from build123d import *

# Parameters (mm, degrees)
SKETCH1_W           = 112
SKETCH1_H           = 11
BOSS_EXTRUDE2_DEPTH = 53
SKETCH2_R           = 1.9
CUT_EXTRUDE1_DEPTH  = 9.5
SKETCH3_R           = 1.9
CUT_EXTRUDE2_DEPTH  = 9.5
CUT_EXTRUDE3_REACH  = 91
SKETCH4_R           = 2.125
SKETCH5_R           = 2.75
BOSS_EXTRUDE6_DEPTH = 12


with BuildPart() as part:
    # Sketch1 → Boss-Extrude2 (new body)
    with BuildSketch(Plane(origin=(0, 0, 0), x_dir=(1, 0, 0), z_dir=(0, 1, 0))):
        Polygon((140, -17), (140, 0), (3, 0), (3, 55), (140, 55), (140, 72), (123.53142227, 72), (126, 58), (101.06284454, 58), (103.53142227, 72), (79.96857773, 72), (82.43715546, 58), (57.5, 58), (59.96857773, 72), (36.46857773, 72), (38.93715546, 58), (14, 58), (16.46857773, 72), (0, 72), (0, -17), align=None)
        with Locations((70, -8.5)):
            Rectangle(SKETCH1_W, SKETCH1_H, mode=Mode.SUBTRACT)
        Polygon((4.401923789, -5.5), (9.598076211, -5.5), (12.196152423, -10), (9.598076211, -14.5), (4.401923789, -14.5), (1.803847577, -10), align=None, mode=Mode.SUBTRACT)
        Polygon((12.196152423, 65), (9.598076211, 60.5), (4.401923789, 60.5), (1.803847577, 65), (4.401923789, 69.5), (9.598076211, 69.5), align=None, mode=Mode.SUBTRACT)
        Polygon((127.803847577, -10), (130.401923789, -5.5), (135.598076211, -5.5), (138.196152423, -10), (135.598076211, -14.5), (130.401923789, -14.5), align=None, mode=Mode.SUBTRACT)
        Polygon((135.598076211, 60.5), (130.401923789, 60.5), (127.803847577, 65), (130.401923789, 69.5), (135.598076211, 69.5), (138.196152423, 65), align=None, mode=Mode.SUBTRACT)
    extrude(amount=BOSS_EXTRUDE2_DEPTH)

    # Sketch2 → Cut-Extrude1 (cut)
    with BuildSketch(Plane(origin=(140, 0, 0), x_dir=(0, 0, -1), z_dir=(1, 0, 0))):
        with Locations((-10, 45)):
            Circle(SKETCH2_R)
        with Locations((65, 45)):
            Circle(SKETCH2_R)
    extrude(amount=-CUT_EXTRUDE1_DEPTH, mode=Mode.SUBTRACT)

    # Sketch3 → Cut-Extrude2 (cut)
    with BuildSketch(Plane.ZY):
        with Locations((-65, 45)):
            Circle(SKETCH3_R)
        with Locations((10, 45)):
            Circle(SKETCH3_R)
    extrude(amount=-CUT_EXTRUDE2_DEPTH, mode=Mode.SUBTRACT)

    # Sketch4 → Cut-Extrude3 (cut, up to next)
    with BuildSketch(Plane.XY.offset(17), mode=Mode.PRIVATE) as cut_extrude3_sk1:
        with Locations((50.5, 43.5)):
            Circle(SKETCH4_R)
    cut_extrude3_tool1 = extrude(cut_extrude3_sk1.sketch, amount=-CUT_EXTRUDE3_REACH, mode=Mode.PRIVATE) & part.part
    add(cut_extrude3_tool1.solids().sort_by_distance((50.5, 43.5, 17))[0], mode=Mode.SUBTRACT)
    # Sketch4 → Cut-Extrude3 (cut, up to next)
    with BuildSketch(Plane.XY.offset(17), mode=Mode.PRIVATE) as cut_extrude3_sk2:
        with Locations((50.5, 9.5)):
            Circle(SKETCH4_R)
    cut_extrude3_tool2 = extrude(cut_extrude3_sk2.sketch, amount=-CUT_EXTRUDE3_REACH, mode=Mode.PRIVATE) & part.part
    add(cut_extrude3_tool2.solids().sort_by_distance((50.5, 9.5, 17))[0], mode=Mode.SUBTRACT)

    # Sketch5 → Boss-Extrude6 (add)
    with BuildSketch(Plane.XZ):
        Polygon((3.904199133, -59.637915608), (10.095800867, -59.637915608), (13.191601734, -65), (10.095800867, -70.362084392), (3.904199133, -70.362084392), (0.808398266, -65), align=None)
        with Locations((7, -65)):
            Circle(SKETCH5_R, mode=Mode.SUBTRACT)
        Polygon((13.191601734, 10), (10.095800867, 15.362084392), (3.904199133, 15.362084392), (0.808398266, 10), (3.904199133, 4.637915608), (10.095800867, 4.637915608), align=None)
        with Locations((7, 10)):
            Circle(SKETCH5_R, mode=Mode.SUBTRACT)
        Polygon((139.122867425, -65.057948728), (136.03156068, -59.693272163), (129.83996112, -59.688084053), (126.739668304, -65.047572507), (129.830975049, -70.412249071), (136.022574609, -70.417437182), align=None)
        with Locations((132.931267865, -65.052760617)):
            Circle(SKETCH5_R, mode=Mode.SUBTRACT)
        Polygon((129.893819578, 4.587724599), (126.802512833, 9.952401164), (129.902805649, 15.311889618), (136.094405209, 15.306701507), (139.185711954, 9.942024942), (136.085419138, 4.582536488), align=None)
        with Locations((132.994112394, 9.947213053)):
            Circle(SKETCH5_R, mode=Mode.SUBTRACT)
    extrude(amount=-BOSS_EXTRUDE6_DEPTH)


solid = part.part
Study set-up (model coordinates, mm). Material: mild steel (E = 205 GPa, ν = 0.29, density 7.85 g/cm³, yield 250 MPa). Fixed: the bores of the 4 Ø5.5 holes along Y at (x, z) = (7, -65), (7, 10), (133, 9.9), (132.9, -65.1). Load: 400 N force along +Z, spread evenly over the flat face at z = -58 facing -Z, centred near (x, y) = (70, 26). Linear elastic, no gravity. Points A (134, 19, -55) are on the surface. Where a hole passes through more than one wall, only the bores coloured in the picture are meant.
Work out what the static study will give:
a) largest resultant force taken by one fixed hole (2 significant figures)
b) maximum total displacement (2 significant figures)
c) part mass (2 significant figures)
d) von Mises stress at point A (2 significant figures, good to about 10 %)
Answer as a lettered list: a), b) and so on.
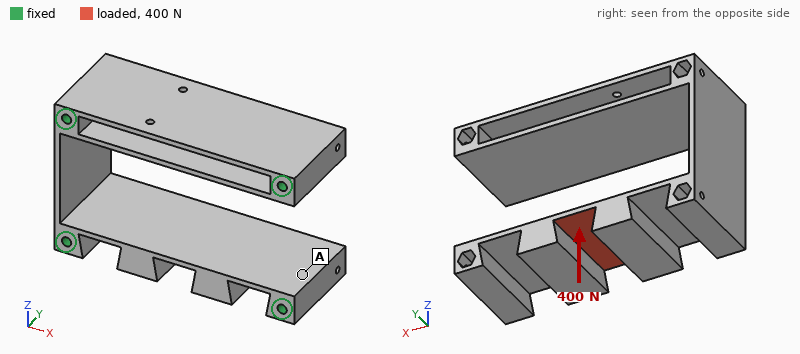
a) 280 N
b) 0.11 mm
c) 1.0 kg
d) 7.4 MPa
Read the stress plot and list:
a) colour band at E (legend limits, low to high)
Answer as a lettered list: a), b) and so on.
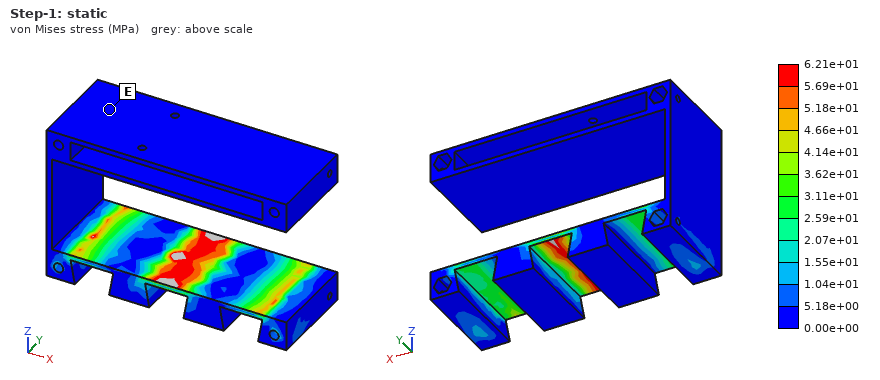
a) 0.00e+00 to 5.18e+00 MPa
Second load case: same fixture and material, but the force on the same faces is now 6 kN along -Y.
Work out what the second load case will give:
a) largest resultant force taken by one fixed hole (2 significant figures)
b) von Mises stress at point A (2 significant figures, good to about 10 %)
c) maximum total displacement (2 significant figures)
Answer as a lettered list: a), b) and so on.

a) 3.5 kN
b) 16 MPa
c) 49 µm
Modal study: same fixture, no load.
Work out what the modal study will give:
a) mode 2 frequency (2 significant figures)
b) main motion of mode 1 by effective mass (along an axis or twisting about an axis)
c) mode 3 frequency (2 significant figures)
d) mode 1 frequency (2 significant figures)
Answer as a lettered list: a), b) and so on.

a) 1200 Hz
b) along Z
c) 1200 Hz
d) 710 Hz
